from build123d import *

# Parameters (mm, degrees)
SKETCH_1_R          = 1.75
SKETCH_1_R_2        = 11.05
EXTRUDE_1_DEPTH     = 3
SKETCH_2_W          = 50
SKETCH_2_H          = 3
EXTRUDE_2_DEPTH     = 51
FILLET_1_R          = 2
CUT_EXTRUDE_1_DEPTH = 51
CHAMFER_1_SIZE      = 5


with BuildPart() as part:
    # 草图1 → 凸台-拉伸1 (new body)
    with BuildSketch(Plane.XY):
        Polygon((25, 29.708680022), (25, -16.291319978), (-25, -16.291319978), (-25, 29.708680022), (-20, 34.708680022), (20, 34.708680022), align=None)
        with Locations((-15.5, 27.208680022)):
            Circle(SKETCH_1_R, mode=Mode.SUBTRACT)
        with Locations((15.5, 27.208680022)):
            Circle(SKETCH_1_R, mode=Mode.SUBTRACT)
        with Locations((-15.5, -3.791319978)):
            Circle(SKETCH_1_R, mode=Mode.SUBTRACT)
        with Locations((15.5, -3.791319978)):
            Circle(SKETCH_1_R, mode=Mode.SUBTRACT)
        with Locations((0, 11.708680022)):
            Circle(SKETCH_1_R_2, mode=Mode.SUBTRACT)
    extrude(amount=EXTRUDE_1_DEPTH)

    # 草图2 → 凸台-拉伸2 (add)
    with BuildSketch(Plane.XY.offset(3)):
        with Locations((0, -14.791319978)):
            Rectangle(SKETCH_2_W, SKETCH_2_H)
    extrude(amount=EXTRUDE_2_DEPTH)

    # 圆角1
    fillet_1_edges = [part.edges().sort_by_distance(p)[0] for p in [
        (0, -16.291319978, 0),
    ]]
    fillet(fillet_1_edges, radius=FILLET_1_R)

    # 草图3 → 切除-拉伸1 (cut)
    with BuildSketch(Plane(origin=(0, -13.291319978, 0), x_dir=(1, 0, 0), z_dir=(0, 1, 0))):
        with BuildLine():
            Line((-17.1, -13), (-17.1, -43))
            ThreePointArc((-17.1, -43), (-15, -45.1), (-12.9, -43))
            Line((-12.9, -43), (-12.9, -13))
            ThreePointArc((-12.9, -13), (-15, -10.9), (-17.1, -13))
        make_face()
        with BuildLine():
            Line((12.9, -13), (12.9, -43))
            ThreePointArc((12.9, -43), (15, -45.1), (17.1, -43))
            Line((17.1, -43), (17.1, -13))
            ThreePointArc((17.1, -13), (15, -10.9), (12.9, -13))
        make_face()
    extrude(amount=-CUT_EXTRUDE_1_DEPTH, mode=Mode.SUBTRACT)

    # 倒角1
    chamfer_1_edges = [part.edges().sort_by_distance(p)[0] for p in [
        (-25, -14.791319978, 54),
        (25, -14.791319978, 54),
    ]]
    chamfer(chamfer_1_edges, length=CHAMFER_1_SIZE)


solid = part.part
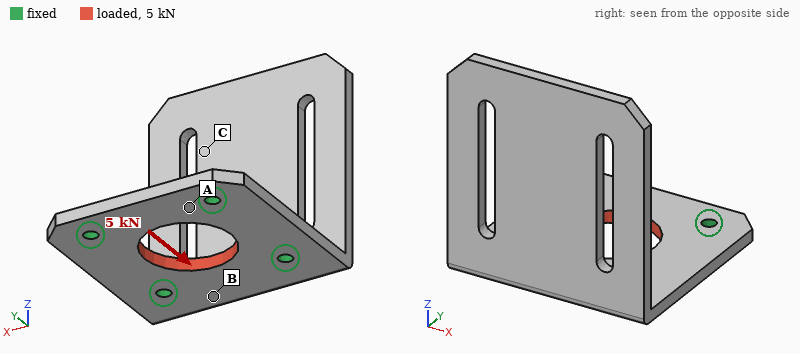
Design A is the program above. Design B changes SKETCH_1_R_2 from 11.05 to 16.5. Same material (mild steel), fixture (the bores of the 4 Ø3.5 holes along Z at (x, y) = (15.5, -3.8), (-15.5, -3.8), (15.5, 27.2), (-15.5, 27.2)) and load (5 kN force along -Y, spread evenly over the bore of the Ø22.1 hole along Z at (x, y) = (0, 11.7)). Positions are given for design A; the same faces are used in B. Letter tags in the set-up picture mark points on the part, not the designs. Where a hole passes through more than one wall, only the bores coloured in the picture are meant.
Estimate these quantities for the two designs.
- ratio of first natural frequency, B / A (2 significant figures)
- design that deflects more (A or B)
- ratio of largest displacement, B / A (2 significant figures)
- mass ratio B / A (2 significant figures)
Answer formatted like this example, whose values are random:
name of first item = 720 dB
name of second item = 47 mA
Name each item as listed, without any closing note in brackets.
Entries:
ratio of first natural frequency, B / A = 0.97
design that deflects more = B
ratio of largest displacement, B / A = 1.4
mass ratio B / A = 0.89
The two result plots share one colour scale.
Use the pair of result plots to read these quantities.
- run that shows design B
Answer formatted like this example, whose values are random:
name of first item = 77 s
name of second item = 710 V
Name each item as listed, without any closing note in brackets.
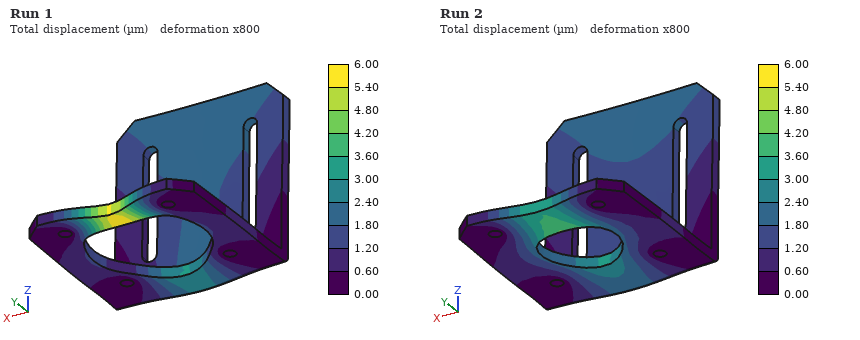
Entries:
run that shows design B = Run 1
